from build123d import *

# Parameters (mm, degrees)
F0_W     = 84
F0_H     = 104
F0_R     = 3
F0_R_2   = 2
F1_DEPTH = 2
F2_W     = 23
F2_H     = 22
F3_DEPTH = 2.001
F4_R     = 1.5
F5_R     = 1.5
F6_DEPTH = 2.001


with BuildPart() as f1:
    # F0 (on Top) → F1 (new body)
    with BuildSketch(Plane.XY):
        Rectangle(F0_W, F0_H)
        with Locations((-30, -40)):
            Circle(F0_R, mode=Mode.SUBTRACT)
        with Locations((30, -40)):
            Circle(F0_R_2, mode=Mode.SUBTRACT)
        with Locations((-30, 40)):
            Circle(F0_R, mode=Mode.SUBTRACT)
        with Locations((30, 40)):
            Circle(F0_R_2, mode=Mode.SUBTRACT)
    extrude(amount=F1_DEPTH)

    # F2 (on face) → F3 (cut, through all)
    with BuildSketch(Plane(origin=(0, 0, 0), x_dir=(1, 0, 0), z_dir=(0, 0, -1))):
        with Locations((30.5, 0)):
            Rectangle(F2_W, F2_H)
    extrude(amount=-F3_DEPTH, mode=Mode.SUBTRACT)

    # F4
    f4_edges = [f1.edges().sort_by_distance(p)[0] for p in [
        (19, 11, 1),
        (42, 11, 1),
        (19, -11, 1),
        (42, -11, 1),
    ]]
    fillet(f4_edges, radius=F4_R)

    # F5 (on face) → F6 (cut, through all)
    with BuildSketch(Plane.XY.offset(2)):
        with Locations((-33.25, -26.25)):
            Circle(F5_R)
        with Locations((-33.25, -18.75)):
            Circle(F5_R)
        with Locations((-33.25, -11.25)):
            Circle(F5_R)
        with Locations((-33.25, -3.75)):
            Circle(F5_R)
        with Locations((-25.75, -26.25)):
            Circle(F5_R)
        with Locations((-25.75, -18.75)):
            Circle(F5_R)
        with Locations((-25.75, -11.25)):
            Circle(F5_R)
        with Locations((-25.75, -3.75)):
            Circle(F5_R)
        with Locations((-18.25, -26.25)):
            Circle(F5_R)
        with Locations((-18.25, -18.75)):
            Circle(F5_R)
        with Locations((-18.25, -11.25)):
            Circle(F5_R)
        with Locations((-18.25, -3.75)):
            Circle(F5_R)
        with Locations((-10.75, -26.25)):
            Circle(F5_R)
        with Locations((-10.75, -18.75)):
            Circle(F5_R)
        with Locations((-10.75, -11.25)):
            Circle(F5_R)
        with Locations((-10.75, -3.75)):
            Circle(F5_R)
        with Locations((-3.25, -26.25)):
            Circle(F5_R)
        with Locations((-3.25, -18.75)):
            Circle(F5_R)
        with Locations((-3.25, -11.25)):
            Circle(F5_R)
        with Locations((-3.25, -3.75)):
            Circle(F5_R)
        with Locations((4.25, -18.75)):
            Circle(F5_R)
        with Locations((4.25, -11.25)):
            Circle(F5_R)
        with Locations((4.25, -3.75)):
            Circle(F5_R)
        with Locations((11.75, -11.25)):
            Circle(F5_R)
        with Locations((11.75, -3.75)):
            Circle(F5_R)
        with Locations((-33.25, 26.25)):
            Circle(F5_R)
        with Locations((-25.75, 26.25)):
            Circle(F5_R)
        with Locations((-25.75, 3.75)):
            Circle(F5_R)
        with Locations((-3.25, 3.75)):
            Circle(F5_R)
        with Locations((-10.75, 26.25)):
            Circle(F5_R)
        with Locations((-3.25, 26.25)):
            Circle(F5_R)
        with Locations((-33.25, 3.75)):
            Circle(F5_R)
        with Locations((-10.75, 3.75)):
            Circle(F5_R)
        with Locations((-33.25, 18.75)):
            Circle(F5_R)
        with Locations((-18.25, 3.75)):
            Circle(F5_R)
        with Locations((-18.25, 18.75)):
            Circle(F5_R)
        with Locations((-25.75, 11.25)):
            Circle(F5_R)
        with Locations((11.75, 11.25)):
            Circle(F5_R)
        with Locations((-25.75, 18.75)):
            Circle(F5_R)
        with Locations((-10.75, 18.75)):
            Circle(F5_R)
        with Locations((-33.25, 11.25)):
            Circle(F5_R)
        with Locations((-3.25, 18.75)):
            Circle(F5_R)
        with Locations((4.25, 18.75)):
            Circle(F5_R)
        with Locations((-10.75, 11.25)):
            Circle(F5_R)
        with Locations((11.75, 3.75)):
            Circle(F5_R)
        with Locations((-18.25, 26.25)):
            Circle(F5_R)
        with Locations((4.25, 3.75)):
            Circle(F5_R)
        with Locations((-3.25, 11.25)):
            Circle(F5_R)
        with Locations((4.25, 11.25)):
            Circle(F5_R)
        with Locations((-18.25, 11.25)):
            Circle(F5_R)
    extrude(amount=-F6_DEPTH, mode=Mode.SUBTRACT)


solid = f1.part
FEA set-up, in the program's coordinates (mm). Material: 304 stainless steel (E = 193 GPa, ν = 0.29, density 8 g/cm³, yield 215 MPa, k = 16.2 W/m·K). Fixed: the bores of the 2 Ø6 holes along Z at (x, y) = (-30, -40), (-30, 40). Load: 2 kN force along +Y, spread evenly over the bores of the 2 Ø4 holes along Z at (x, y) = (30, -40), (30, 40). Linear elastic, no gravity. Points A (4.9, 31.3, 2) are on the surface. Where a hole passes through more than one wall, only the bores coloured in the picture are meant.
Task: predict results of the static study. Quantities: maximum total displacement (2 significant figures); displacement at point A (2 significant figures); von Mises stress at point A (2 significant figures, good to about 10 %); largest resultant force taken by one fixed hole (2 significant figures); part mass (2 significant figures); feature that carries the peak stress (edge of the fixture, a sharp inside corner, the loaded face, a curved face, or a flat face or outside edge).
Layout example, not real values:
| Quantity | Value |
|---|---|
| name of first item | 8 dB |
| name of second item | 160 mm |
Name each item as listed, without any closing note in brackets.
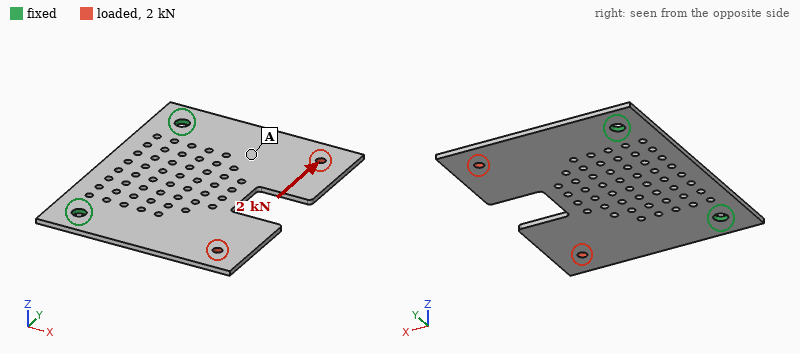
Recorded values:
| Quantity | Value |
|---|---|
| maximum total displacement | 28 µm |
| displacement at point A | 11 µm |
| von Mises stress at point A | 17 MPa |
| largest resultant force taken by one fixed hole | 1.7 kN |
| part mass | 120 g |
| feature that carries the peak stress | a curved face |
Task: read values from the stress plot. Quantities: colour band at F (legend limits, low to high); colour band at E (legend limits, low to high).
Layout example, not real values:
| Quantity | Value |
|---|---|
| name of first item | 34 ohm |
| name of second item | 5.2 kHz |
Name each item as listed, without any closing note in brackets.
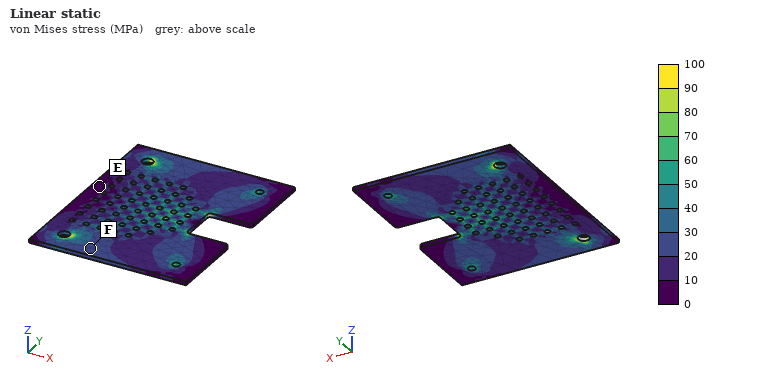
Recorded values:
| Quantity | Value |
|---|---|
| colour band at F | 20 to 30 MPa |
| colour band at E | 0 to 10 MPa |
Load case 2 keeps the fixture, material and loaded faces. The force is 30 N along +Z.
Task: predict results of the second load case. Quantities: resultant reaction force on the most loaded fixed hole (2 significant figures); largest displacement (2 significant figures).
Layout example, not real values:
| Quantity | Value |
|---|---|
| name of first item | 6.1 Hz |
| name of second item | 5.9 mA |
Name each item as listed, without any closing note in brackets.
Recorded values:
| Quantity | Value |
|---|---|
| resultant reaction force on the most loaded fixed hole | 15 N |
| largest displacement | 0.27 mm |
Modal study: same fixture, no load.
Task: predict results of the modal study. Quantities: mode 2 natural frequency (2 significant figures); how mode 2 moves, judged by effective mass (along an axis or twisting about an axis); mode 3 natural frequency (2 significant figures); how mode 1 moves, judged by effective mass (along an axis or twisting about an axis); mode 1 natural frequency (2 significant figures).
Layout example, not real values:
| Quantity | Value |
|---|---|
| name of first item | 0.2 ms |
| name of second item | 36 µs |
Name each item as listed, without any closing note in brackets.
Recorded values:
| Quantity | Value |
|---|---|
| mode 2 natural frequency | 500 Hz |
| how mode 2 moves, judged by effective mass | twisting about X |
| mode 3 natural frequency | 1100 Hz |
| how mode 1 moves, judged by effective mass | along Z |
| mode 1 natural frequency | 290 Hz |
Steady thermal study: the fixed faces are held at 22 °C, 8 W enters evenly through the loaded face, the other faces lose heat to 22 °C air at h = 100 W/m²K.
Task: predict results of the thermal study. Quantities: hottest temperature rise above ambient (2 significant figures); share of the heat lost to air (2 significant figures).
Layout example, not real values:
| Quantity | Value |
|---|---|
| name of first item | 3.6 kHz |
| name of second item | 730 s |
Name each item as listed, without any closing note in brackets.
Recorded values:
| Quantity | Value |
|---|---|
| hottest temperature rise above ambient | 48 K |
| share of the heat lost to air | 99 % |
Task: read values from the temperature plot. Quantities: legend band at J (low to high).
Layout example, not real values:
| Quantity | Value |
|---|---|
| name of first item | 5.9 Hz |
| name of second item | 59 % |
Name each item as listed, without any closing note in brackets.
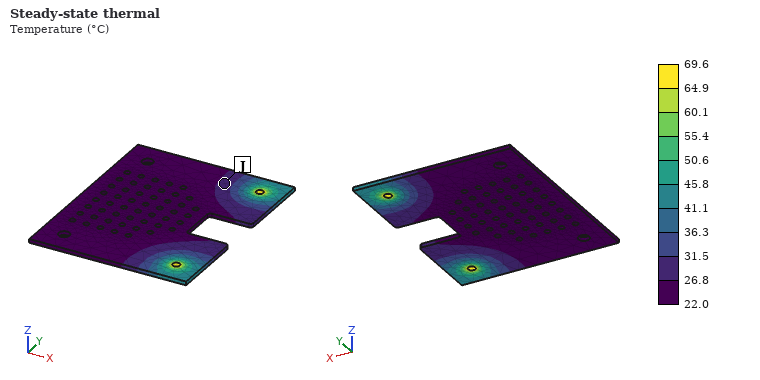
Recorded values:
| Quantity | Value |
|---|---|
| legend band at J | 26.8 to 31.5 °C |
